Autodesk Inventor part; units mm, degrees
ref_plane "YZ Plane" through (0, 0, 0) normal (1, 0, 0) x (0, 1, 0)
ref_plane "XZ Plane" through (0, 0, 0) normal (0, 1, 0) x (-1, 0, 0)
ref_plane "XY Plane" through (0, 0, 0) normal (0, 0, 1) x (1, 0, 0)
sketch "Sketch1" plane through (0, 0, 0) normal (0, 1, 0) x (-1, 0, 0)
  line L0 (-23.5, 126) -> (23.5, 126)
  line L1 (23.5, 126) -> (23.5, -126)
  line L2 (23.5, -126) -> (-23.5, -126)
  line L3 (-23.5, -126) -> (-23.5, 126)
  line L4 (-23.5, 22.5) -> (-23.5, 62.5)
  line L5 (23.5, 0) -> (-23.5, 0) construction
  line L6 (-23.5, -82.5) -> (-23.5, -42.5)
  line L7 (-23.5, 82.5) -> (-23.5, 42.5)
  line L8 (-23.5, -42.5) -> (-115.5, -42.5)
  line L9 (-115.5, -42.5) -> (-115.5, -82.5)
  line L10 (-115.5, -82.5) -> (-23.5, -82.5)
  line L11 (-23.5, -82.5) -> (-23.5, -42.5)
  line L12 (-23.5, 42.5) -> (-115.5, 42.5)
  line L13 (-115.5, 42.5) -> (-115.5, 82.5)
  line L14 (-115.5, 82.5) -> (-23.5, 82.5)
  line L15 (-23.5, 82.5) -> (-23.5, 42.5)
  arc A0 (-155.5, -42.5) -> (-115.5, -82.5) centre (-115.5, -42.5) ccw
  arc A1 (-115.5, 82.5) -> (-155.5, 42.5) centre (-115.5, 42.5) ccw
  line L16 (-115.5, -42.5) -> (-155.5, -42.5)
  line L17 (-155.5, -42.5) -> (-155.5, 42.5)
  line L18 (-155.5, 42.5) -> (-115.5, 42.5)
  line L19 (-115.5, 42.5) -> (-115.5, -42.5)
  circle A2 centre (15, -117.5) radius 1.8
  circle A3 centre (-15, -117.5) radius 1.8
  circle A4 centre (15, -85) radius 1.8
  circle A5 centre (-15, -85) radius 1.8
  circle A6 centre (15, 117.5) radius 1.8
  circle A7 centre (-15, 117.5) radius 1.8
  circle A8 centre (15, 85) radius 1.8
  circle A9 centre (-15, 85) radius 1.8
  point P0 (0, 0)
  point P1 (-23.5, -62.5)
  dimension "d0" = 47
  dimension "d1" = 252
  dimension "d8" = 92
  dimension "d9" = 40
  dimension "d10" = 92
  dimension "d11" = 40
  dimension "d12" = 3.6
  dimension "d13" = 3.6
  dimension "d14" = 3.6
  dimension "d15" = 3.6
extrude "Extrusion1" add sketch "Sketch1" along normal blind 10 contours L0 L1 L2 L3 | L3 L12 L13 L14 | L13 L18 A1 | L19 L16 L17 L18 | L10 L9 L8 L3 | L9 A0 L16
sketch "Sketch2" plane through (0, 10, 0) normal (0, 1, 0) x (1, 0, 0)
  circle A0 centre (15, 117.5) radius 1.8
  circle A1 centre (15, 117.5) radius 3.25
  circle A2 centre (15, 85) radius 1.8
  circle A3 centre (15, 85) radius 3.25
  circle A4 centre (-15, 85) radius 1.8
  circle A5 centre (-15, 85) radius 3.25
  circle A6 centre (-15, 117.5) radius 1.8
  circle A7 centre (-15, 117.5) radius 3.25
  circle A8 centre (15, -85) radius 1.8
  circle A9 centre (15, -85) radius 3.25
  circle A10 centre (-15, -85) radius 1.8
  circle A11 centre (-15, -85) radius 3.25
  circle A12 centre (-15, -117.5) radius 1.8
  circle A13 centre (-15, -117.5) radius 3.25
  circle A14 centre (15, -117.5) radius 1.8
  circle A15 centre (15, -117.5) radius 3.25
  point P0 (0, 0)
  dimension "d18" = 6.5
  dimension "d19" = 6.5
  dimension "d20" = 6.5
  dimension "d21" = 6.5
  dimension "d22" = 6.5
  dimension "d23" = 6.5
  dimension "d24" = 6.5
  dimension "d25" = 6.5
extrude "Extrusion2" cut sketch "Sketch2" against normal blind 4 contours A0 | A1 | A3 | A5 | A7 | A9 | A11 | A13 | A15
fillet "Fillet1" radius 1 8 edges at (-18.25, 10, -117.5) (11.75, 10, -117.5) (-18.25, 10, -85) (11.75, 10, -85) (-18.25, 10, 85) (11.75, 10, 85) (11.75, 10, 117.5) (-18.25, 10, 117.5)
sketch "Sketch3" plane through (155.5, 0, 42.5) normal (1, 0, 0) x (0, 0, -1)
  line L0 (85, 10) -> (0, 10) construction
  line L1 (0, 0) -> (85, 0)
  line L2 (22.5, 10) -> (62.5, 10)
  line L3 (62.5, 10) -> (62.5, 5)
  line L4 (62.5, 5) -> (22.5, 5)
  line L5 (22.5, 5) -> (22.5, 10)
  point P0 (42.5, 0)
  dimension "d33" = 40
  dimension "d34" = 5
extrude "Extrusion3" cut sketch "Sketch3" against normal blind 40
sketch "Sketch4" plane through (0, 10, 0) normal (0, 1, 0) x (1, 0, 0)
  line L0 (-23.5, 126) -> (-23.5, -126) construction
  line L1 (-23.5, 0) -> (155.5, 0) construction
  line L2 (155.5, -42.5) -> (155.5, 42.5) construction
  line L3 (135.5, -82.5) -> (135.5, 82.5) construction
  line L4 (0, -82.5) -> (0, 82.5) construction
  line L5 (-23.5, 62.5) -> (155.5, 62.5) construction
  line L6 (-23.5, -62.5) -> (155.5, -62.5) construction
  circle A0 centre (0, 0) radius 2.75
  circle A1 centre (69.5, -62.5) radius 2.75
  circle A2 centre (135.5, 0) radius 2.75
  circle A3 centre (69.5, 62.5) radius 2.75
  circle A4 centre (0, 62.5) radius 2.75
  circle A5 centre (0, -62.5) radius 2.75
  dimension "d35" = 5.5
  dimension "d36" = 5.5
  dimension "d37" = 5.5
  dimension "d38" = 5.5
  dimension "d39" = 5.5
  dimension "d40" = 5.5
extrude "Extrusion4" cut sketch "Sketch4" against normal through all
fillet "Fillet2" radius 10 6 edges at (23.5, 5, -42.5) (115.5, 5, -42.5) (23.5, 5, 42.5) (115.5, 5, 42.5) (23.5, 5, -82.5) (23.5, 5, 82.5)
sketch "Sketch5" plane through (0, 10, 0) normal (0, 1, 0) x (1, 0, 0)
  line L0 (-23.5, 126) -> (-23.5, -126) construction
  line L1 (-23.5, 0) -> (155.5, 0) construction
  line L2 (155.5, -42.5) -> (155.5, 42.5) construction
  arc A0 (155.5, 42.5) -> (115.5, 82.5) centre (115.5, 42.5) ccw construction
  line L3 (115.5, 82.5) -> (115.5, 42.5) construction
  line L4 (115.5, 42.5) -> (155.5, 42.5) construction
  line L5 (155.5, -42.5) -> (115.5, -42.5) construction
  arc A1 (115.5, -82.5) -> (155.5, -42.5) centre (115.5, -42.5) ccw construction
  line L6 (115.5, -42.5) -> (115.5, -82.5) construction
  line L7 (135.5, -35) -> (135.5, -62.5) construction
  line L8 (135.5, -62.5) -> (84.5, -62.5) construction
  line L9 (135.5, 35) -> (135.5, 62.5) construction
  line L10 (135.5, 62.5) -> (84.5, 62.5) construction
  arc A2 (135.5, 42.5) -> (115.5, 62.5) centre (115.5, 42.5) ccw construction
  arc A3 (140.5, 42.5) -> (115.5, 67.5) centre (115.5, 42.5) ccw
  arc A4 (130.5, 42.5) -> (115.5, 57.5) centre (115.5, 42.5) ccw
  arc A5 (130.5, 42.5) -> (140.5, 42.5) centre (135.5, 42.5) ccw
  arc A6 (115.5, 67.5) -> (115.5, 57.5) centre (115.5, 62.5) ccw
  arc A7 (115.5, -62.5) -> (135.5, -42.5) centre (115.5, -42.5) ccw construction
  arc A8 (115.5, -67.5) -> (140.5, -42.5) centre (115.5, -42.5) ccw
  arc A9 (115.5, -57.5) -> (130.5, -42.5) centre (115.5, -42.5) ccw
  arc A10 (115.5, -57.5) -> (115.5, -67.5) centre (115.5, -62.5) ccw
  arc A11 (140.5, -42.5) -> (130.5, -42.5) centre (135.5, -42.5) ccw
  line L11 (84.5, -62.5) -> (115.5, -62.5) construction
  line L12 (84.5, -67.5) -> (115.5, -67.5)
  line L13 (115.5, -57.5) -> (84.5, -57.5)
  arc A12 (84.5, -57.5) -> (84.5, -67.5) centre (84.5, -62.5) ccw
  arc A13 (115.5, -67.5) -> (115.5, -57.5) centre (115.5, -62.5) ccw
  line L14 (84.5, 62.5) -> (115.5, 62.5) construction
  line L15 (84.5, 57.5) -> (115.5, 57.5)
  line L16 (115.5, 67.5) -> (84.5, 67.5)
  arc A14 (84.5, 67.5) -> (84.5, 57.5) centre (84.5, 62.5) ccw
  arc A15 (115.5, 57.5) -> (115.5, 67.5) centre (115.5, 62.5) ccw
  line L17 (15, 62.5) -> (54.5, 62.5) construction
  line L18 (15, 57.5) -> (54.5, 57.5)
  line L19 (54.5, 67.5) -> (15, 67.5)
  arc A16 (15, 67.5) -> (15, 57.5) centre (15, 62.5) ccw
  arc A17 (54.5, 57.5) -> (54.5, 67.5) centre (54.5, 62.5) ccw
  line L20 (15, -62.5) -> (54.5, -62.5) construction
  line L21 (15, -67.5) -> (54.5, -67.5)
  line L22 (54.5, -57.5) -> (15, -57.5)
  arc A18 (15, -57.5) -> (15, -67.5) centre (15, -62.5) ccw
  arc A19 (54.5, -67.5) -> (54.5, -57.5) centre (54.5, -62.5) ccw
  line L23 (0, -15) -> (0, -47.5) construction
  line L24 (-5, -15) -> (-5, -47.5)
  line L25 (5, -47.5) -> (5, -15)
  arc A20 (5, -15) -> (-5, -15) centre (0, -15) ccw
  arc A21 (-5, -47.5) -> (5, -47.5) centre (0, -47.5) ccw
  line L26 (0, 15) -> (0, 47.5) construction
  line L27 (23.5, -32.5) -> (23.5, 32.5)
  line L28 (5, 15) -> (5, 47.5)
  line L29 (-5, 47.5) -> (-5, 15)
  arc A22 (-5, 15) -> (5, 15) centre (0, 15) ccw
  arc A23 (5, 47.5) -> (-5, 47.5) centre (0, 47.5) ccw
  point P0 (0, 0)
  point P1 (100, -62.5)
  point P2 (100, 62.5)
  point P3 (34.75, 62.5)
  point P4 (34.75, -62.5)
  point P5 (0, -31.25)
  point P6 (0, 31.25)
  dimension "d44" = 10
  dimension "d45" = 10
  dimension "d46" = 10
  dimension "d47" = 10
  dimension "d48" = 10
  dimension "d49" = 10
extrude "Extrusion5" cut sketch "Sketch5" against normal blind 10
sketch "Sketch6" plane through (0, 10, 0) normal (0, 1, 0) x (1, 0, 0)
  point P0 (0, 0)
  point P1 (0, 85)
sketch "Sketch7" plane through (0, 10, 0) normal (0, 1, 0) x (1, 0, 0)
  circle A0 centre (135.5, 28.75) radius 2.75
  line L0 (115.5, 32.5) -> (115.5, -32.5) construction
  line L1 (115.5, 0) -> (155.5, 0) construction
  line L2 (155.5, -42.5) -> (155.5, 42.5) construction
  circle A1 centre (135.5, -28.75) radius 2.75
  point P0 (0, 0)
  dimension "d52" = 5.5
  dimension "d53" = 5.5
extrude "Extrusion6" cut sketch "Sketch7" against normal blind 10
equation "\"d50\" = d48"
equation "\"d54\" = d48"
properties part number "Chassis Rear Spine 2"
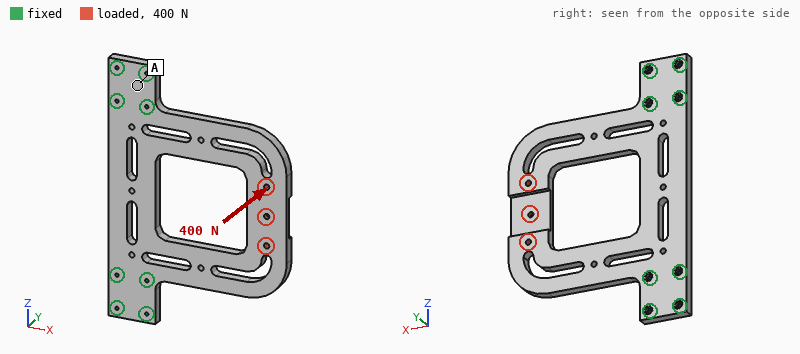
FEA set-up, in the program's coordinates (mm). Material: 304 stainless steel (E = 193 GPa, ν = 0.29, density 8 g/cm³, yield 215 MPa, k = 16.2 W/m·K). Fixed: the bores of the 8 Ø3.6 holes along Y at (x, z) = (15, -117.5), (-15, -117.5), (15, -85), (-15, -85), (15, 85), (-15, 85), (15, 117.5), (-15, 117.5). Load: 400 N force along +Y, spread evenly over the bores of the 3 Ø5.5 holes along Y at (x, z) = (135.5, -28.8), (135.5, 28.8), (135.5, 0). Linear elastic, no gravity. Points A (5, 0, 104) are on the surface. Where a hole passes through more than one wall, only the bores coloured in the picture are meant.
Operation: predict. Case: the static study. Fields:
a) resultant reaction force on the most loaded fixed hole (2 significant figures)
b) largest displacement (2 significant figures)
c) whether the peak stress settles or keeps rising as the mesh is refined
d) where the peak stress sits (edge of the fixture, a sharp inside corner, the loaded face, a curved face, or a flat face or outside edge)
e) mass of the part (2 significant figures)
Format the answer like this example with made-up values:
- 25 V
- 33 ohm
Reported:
- 1.1 kN
- 0.42 mm
- keeps rising
- edge of the fixture
- 1.7 kg
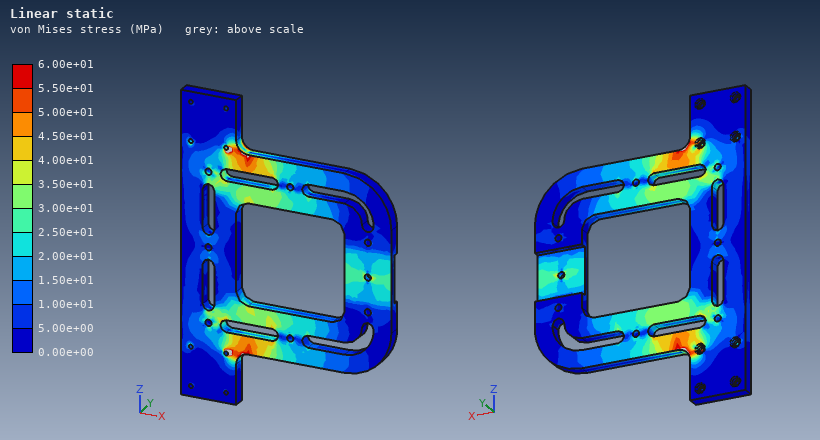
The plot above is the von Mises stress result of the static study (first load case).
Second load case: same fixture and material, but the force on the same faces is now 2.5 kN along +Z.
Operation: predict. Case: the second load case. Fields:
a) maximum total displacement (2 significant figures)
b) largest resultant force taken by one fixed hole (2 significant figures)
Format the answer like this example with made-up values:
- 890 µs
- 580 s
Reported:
- 55 µm
- 1.6 kN
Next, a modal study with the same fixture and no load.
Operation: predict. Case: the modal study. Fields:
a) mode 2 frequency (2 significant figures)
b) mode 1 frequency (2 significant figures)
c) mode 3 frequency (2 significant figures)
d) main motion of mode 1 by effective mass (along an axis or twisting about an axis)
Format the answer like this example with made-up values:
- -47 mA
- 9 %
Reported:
- 660 Hz
- 280 Hz
- 1400 Hz
- along Y
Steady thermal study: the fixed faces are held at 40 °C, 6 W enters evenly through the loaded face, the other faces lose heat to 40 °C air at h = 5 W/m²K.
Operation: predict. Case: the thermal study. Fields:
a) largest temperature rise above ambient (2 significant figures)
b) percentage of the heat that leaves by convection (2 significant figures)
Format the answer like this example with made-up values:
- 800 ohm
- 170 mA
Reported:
- 46 K
- 71 %
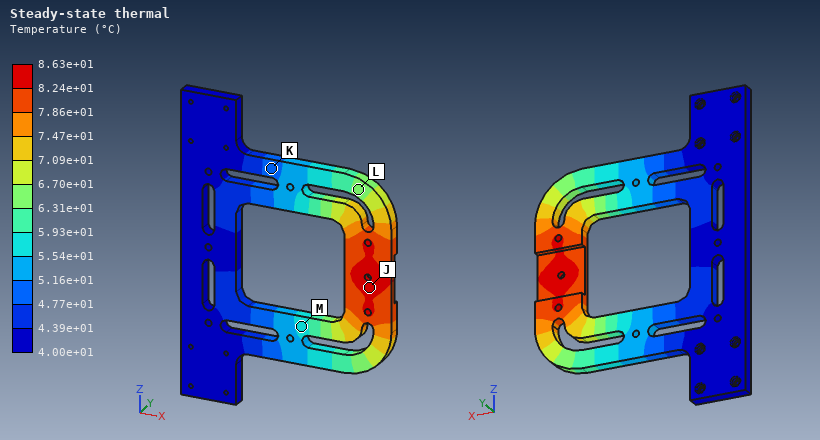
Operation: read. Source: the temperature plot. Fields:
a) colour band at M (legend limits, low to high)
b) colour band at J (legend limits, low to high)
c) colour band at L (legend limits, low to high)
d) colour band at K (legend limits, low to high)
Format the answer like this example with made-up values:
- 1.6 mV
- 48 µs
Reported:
- 5.54e+01 to 5.93e+01 °C
- 8.24e+01 to 8.63e+01 °C
- 6.31e+01 to 6.70e+01 °C
- 4.77e+01 to 5.16e+01 °C
